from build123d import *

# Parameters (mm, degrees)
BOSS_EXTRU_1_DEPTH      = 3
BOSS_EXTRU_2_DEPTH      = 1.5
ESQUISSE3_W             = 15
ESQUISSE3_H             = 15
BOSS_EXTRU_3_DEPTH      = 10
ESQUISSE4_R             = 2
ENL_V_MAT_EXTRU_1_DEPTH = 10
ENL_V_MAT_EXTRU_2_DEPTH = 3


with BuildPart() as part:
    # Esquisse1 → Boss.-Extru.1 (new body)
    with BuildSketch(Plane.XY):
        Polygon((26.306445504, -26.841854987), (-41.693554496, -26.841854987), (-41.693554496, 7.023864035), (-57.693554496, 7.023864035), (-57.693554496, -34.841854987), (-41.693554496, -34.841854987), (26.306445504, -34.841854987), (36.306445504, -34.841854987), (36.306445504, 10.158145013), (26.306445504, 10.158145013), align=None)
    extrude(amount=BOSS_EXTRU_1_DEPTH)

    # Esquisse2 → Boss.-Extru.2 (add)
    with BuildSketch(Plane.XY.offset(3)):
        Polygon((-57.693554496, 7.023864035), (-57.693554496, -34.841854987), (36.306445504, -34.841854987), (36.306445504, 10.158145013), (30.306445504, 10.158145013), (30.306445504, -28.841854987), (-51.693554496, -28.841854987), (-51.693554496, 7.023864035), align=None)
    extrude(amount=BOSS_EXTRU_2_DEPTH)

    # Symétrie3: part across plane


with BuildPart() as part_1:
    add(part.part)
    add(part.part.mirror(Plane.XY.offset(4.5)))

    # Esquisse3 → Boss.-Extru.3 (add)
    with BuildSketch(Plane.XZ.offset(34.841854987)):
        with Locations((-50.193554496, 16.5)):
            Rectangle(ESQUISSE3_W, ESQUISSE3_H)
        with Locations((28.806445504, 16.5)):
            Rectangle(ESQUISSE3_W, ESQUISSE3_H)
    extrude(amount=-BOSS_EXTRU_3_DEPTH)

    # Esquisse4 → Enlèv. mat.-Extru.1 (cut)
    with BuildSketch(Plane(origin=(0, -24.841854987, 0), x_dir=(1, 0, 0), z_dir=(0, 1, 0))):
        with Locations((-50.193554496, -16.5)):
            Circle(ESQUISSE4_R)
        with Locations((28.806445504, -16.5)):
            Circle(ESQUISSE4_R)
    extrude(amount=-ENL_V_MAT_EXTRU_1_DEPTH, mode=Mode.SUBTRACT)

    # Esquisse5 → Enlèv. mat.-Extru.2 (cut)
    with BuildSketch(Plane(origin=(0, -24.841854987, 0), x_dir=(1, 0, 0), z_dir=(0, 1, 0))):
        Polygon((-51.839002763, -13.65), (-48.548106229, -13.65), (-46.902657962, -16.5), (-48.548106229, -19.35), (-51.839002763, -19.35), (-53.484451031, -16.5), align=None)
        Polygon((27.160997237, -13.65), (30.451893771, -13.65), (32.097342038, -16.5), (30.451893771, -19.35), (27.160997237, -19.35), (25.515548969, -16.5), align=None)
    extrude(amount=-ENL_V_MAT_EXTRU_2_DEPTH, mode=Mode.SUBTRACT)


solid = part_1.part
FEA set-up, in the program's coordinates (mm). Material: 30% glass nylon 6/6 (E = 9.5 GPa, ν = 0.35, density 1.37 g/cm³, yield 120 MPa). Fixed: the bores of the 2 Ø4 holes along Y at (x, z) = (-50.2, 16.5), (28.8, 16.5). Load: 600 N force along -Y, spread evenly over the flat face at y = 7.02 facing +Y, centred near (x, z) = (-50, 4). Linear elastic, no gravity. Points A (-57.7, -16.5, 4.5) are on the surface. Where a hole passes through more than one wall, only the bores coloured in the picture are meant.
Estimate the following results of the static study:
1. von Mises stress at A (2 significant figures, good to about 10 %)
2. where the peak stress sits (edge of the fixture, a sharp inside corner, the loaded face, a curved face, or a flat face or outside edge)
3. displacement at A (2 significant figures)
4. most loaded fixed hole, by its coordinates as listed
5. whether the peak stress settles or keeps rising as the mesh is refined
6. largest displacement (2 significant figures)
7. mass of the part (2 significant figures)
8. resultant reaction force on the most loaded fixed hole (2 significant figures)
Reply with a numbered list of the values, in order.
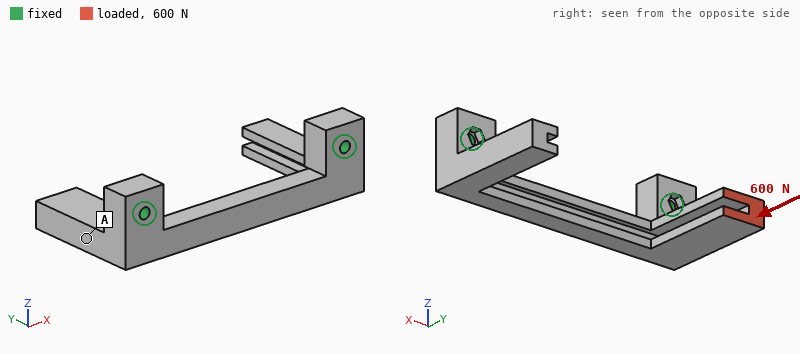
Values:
1. 5.2 MPa
2. edge of the fixture
3. 0.13 mm
4. (-50.2, 16.5)
5. keeps rising
6. 0.30 mm
7. 24 g
8. 600 N
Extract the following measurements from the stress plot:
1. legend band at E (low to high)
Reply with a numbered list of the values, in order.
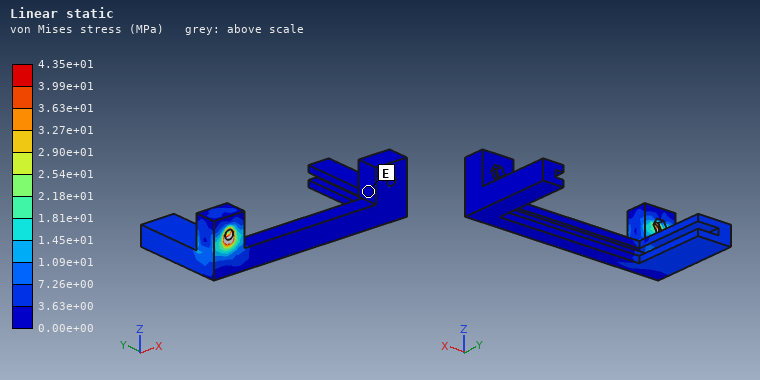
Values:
1. 0.00e+00 to 3.63e+00 MPa
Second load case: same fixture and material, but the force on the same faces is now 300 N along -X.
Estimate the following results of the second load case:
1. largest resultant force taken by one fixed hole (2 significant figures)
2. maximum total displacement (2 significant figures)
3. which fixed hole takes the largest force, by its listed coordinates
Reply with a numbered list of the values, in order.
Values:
1. 220 N
2. 0.71 mm
3. (-50.2, 16.5)
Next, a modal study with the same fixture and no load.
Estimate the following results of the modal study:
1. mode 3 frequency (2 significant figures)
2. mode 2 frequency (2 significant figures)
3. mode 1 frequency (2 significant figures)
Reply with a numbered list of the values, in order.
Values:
1. 1900 Hz
2. 1800 Hz
3. 1800 Hz
